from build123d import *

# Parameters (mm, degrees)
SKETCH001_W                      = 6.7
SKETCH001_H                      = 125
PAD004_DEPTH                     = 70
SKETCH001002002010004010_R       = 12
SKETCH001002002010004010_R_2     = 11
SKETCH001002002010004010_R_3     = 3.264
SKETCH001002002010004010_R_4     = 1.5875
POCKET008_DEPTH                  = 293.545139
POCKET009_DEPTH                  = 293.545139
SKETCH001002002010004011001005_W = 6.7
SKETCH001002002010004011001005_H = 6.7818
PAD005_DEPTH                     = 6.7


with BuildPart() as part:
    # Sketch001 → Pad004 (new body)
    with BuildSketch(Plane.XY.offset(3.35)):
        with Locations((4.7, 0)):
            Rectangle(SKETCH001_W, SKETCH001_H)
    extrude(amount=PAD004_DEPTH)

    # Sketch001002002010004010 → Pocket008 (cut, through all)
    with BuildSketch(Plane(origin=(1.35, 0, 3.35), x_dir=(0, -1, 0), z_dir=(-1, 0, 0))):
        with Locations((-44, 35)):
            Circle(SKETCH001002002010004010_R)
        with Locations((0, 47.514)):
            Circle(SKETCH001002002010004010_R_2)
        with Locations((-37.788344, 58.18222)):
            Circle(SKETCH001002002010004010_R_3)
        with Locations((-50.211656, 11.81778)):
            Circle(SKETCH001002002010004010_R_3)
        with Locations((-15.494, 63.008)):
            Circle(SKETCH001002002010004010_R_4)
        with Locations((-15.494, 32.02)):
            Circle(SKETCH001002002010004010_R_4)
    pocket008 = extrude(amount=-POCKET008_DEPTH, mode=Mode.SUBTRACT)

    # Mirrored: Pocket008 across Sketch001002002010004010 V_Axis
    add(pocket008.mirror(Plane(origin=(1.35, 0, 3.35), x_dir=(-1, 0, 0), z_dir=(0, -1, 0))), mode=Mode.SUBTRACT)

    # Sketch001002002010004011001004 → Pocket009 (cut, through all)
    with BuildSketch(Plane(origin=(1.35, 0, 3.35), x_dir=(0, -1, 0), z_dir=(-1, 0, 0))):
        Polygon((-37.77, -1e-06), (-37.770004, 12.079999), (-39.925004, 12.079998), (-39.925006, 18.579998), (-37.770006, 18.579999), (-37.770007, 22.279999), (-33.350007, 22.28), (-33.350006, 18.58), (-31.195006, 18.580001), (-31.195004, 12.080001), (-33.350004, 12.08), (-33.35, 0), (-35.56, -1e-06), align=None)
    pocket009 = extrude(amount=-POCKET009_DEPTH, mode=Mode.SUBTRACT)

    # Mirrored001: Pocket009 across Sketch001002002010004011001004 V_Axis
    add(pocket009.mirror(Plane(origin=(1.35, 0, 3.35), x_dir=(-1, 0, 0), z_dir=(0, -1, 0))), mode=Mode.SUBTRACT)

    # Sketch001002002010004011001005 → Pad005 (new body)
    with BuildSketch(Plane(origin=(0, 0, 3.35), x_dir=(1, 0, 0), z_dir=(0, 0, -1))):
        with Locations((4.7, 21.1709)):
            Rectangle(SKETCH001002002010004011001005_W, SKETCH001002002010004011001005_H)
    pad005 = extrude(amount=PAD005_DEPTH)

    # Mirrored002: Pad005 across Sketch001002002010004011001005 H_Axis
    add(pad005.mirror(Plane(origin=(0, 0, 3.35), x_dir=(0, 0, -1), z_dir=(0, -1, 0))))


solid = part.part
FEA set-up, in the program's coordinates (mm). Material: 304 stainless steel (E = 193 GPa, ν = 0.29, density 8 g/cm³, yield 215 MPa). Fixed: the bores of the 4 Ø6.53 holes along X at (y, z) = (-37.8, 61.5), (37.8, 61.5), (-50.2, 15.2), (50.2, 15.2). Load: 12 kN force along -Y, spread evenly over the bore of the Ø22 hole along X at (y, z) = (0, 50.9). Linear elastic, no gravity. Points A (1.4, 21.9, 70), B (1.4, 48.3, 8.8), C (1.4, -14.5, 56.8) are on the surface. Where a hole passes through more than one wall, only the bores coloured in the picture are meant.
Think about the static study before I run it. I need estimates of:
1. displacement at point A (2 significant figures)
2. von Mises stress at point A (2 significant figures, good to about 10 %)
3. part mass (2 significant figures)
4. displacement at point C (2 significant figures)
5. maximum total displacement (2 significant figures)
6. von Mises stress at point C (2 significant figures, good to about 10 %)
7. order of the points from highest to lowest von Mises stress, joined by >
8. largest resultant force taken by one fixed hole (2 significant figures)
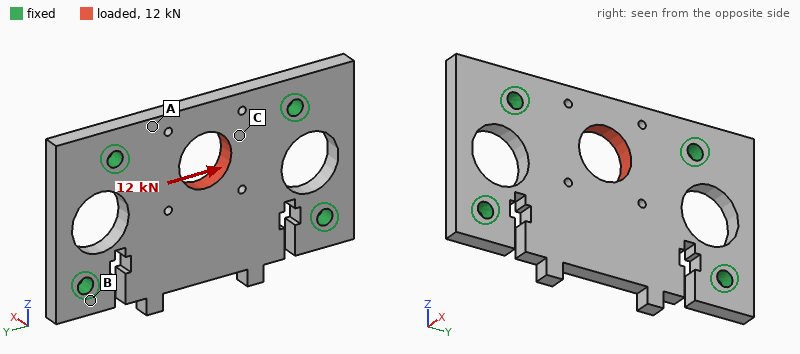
2.1 µm
19 MPa
380 g
4.1 µm
7.3 µm
29 MPa
C > A > B
5.1 kN
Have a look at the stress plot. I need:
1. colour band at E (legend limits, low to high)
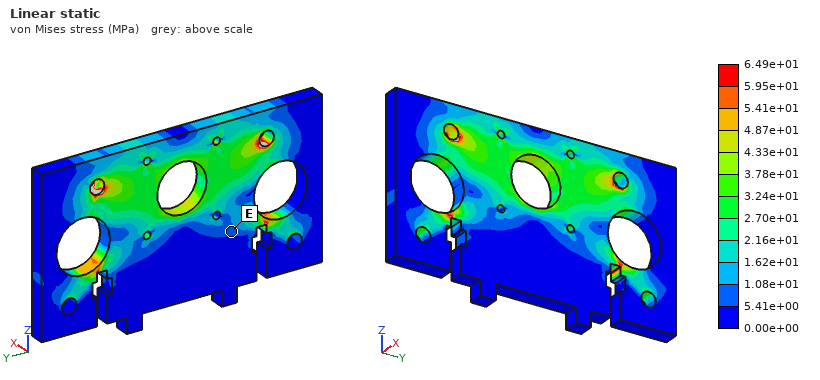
5.41e+00 to 1.08e+01 MPa
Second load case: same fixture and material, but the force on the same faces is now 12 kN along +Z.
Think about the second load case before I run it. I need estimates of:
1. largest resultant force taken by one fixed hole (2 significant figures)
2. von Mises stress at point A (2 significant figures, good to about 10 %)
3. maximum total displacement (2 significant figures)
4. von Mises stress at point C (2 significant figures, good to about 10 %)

5.7 kN
13 MPa
18 µm
35 MPa
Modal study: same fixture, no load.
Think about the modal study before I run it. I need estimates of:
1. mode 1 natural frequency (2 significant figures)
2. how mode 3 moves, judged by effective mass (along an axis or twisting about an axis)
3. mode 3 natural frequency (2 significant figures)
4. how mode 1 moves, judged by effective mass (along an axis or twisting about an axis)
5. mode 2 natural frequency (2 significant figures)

1900 Hz
along X
5700 Hz
along X
5000 Hz
